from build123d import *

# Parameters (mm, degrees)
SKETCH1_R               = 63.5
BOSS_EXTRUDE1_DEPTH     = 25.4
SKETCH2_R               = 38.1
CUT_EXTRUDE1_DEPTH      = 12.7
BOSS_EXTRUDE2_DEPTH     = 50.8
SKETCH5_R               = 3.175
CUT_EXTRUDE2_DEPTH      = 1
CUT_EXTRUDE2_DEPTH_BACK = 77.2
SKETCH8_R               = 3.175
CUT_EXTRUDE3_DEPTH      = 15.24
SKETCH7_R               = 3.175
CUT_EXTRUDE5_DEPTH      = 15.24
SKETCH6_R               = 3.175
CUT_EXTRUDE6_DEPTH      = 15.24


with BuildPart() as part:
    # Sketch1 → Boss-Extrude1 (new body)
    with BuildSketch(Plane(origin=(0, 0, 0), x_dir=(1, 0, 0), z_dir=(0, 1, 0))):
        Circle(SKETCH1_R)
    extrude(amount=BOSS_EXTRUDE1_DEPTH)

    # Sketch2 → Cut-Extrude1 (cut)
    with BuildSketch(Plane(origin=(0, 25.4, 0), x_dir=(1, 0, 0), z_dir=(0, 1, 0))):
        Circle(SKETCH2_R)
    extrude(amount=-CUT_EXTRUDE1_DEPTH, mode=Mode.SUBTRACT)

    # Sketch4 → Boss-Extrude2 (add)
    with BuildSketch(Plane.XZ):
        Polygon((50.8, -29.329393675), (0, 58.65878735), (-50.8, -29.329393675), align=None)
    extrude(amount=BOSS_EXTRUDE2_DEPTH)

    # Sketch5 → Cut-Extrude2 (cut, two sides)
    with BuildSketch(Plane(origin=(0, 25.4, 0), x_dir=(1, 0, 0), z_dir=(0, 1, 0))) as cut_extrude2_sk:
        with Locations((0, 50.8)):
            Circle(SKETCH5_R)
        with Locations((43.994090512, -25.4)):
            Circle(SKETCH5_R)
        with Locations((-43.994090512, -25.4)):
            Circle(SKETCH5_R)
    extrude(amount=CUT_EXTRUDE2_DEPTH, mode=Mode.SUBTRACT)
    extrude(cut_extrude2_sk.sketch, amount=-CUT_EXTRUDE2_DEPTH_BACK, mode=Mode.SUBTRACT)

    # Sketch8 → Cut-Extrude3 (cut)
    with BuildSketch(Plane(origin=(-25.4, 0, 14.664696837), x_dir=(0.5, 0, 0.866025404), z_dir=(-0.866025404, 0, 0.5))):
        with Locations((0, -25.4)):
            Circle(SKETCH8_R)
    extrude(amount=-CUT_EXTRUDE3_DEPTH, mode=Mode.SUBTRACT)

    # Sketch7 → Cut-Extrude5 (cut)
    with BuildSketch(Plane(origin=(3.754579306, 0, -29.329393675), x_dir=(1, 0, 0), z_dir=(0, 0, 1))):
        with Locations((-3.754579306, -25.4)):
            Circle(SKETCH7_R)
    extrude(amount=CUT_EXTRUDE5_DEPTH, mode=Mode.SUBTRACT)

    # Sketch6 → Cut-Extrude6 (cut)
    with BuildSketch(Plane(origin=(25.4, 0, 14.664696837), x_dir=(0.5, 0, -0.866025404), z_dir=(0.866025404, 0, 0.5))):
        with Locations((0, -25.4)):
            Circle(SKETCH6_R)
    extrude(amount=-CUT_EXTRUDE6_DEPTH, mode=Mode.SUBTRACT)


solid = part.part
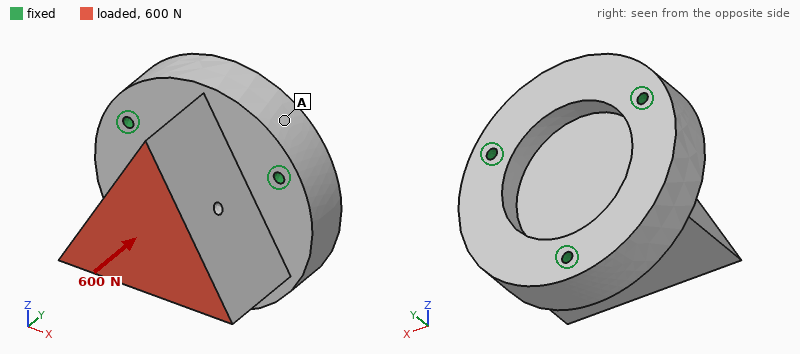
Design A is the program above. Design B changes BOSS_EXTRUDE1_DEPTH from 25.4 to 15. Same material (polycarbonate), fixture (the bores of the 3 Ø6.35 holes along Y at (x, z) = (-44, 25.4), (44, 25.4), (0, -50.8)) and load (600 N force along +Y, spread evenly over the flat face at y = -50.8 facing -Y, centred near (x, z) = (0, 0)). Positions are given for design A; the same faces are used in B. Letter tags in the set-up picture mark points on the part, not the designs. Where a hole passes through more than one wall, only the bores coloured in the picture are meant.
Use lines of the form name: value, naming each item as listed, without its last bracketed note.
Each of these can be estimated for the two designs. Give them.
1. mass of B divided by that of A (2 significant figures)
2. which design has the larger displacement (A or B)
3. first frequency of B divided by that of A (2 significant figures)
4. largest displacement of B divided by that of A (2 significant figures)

mass of B divided by that of A: 0.83
which design has the larger displacement: B
first frequency of B divided by that of A: 0.76
largest displacement of B divided by that of A: 1.9
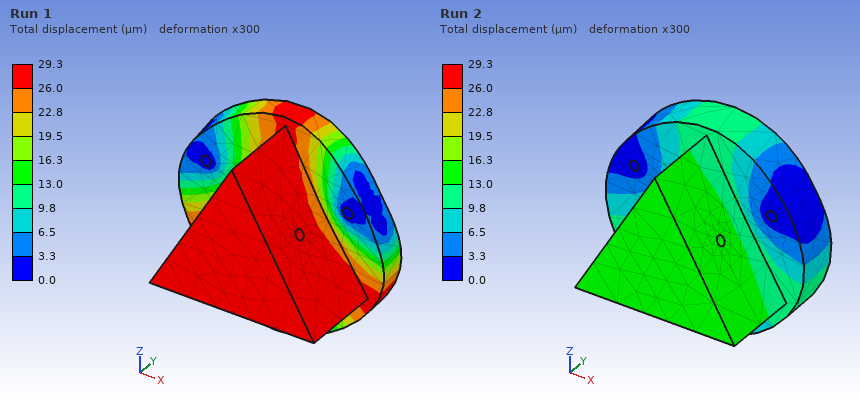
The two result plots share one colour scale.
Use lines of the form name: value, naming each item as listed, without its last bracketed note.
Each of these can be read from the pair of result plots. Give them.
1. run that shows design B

run that shows design B: Run 1
